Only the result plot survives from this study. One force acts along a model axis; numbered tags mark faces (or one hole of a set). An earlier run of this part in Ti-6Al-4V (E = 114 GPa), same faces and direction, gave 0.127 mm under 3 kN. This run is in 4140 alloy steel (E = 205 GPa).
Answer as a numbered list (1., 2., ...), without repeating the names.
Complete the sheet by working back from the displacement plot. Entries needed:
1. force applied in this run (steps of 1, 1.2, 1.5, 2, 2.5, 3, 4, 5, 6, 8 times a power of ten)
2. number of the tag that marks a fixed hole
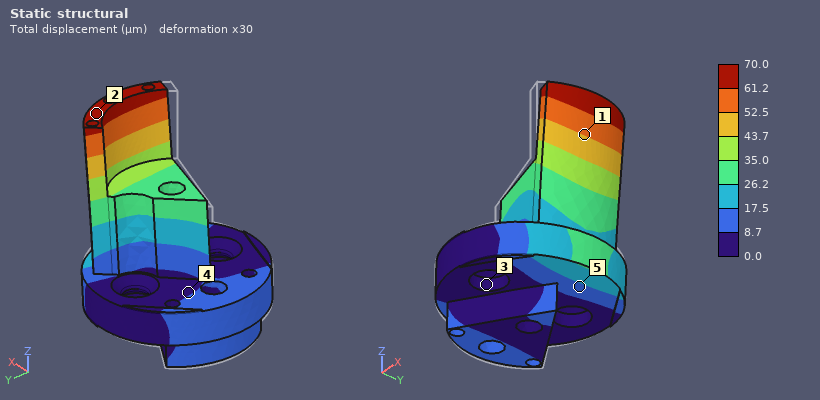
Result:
1. 3 kN
2. 3
